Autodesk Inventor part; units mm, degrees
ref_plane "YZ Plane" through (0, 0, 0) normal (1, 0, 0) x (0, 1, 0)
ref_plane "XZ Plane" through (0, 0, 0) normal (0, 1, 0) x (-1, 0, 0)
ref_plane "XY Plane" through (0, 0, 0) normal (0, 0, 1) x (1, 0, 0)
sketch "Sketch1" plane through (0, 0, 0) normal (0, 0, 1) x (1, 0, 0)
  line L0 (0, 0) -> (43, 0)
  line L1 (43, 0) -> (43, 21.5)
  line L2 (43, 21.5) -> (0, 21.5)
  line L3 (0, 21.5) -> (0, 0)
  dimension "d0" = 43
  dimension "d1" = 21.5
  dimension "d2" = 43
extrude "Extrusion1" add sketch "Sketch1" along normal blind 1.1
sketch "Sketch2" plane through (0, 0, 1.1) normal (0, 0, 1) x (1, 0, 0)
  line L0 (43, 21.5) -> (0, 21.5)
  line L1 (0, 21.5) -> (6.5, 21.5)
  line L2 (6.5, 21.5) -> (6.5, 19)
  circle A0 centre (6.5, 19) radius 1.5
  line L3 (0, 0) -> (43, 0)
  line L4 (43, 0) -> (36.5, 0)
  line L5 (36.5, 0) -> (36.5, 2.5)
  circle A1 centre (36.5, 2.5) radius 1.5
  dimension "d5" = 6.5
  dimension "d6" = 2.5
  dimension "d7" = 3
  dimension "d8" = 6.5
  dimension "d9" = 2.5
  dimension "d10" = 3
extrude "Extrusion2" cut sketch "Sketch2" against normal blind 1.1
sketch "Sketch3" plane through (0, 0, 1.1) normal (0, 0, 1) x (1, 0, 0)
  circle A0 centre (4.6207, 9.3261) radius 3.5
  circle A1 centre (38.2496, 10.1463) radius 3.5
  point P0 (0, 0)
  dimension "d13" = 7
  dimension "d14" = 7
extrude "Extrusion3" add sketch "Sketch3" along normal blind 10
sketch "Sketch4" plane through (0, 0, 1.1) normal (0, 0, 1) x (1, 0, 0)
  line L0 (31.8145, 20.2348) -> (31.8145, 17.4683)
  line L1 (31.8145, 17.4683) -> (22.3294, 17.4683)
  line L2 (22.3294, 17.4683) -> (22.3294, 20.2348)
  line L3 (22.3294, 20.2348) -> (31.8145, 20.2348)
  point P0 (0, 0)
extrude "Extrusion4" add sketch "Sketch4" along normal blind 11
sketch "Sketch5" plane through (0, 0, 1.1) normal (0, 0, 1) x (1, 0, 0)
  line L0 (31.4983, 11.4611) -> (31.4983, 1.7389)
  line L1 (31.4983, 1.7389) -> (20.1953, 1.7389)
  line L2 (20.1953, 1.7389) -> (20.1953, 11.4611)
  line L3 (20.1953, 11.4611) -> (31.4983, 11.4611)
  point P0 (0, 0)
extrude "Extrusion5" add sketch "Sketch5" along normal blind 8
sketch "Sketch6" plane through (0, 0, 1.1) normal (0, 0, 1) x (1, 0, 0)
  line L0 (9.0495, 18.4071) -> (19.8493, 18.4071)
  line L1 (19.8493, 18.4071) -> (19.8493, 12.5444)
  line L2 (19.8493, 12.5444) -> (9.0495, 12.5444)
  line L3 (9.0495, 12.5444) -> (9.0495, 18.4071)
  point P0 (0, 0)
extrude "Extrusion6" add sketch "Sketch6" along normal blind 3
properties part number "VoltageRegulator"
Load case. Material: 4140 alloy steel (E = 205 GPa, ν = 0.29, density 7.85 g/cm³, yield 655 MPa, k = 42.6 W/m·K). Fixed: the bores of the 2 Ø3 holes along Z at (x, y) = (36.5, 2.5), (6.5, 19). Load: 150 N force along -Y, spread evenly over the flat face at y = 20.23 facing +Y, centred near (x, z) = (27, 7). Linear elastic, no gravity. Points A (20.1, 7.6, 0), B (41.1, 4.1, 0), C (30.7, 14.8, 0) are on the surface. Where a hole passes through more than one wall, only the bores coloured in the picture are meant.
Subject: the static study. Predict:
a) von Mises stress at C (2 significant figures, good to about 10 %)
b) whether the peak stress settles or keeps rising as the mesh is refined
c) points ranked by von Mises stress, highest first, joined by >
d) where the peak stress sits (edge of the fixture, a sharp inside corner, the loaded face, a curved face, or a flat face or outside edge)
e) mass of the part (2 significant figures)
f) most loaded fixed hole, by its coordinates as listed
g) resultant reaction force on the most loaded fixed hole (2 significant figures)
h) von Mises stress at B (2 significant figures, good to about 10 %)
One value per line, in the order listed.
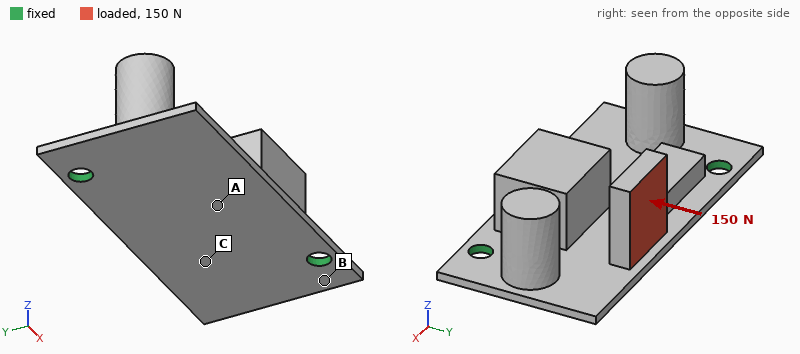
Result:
100 MPa
keeps rising
C > B > A
edge of the fixture
25 g
(36.5, 2.5)
93 N
61 MPa
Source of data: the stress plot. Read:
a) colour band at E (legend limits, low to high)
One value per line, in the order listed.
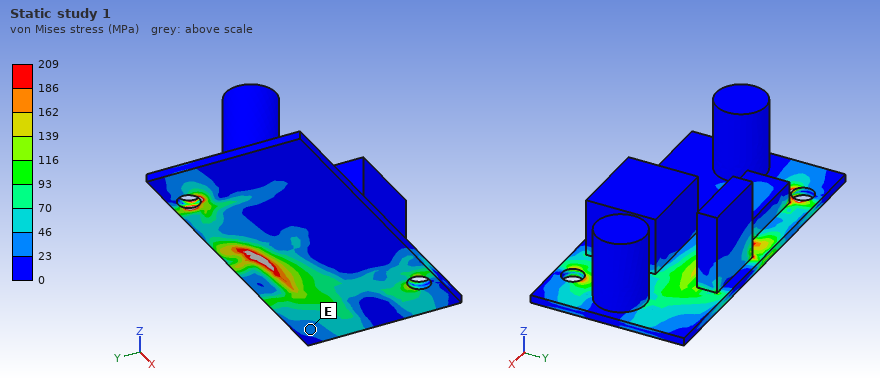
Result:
23 to 46 MPa
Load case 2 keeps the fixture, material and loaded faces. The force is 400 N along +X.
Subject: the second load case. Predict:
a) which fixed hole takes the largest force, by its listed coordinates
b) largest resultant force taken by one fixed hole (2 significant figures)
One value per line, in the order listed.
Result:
(6.5, 19)
290 N
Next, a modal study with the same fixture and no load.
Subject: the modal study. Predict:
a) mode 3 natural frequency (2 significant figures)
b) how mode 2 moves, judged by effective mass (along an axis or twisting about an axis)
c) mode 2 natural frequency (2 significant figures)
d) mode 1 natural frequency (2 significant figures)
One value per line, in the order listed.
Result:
3400 Hz
along Z
2700 Hz
2000 Hz
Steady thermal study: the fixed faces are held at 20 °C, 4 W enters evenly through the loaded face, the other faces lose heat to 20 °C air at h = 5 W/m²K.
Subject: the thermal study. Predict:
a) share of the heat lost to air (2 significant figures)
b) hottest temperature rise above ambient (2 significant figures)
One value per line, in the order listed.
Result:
7.7 %
68 K
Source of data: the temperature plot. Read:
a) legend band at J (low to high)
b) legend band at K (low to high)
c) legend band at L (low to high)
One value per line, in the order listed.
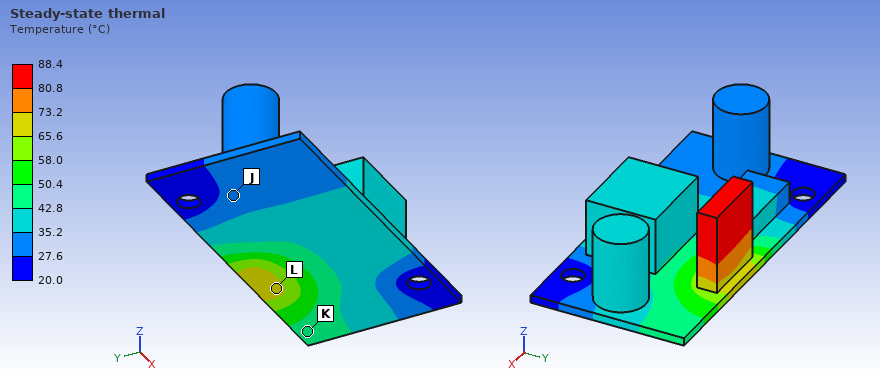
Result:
27.6 to 35.2 °C
42.8 to 50.4 °C
65.6 to 73.2 °C
